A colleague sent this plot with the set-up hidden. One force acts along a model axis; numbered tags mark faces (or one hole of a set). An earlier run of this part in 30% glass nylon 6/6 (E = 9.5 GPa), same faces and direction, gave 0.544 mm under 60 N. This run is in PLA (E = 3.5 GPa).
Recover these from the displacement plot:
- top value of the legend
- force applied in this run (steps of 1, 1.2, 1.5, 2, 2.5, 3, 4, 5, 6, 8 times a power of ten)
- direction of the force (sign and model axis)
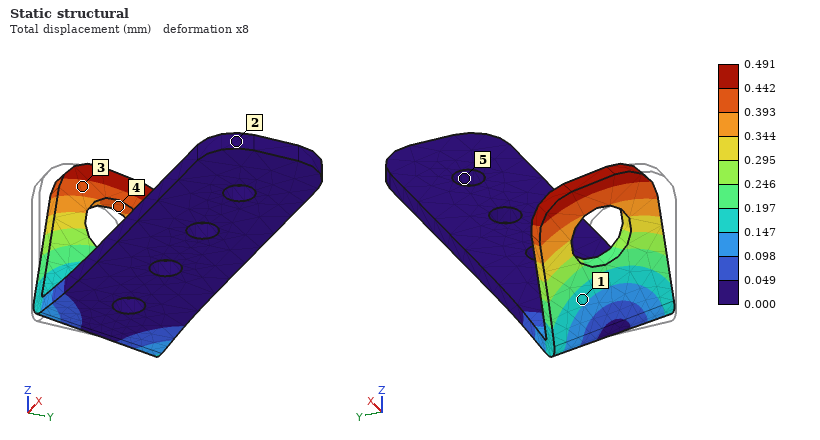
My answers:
0.491 mm
20 N
+Y
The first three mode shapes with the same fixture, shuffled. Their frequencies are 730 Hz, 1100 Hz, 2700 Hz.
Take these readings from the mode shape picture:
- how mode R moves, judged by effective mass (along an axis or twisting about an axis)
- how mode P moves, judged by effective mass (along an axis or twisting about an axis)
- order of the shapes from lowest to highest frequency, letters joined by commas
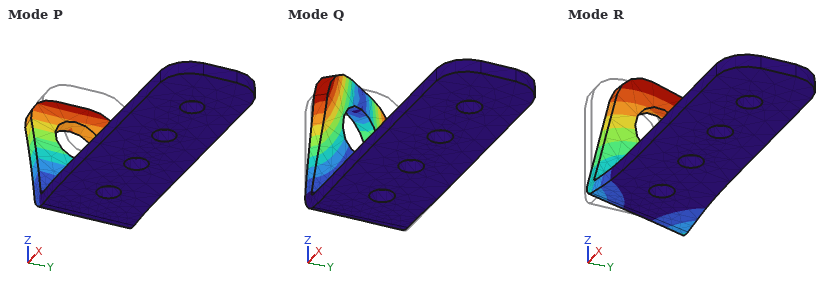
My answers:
along Y
along X
P, R, Q
